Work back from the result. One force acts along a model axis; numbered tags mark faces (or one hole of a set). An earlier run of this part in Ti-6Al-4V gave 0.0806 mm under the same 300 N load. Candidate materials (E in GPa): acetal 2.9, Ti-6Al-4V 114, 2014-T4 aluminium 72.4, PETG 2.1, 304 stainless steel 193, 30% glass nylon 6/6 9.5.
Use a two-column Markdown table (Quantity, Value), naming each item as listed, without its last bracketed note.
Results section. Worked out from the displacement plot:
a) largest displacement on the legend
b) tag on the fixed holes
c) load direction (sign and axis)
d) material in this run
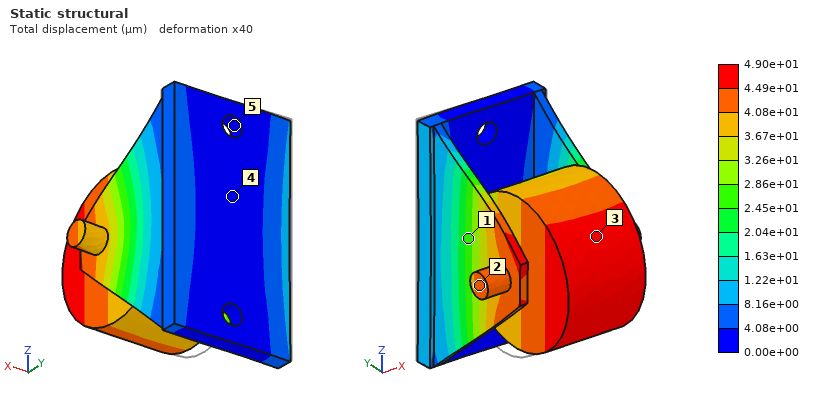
| Quantity | Value |
|---|---|
| largest displacement on the legend | 4.90e+01 µm |
| tag on the fixed holes | 5 |
| load direction | +X |
| material in this run | 304 stainless steel |
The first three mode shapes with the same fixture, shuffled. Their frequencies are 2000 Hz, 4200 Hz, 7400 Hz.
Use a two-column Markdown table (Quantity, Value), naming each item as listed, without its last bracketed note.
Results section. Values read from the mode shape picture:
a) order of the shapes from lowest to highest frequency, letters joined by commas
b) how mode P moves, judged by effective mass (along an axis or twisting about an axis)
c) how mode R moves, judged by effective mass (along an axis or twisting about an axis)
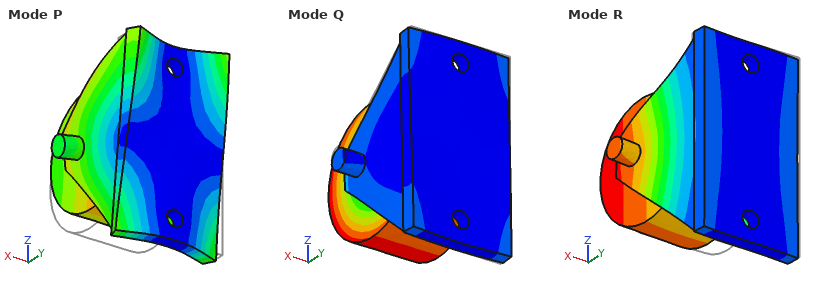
| Quantity | Value |
|---|---|
| order of the shapes from lowest to highest frequency, letters joined by commas | R, Q, P |
| how mode P moves, judged by effective mass | along Z |
| how mode R moves, judged by effective mass | along X |
